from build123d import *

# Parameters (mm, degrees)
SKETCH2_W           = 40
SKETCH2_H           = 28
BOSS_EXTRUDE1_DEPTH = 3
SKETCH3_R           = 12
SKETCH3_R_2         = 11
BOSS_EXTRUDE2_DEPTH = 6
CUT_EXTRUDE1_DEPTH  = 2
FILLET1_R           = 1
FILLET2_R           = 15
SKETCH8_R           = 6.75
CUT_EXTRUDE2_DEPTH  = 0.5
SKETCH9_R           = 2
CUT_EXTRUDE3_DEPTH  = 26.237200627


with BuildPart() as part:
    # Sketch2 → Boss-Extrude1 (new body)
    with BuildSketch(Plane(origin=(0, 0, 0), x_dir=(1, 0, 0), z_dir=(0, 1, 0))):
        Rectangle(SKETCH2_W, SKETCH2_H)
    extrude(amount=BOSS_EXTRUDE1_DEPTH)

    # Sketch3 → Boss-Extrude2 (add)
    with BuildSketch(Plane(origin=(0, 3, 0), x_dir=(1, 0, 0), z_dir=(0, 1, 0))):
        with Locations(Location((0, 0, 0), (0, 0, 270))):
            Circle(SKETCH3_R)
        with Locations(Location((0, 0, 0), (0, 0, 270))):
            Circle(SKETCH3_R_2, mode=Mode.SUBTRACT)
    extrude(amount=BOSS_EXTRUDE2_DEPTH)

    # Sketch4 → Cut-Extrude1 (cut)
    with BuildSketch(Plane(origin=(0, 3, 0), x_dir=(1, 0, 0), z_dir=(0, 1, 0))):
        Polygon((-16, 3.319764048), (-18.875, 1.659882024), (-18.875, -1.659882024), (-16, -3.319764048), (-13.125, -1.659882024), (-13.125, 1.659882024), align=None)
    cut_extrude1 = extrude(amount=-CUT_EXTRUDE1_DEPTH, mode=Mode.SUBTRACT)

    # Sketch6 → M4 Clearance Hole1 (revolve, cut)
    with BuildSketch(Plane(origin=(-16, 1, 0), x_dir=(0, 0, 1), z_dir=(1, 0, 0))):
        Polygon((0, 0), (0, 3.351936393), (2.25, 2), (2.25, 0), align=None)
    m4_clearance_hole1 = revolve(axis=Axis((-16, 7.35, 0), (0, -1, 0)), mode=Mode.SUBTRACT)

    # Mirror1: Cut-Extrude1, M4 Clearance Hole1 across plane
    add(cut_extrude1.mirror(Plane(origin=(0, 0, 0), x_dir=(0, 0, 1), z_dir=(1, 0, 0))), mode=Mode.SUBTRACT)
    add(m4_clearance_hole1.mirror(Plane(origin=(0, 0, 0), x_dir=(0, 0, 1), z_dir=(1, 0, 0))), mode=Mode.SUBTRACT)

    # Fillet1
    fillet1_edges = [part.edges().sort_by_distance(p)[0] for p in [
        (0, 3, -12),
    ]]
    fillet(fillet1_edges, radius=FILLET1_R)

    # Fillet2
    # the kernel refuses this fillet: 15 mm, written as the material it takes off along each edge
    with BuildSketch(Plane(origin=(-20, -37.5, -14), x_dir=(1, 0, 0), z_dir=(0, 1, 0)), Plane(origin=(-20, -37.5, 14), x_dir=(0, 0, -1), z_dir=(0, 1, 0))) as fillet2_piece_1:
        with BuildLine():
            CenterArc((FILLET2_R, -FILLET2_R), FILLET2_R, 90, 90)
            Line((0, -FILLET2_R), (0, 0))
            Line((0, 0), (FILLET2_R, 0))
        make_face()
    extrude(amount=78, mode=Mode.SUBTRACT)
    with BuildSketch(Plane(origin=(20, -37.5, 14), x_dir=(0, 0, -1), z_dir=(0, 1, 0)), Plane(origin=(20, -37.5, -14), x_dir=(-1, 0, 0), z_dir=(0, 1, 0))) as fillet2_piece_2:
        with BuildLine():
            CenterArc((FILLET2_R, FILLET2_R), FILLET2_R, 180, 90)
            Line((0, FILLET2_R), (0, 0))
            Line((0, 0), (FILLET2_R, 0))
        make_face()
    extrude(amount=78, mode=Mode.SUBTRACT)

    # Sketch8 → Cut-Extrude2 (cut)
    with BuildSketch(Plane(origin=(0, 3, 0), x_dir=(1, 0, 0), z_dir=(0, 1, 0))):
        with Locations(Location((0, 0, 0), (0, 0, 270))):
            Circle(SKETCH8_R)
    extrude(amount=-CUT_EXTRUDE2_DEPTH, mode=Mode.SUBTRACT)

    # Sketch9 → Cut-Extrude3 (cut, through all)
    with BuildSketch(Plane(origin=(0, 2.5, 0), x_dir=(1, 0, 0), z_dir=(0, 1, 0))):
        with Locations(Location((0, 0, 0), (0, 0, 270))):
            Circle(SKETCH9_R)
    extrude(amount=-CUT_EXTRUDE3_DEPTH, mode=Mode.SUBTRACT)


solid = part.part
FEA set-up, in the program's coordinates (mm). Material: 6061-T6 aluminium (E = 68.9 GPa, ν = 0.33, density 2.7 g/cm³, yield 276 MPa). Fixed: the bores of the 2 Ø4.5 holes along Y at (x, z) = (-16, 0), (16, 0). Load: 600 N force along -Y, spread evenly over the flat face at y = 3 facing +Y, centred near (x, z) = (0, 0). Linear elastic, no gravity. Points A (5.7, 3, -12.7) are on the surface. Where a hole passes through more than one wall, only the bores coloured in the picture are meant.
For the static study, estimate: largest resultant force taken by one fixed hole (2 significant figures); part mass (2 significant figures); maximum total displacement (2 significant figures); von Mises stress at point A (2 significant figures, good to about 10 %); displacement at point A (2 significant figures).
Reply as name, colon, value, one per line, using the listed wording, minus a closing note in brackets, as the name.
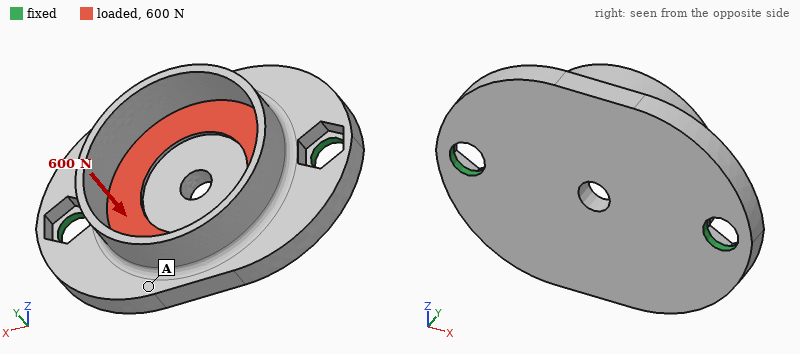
largest resultant force taken by one fixed hole: 450 N
part mass: 8.0 g
maximum total displacement: 44 µm
von Mises stress at point A: 22 MPa
displacement at point A: 31 µm
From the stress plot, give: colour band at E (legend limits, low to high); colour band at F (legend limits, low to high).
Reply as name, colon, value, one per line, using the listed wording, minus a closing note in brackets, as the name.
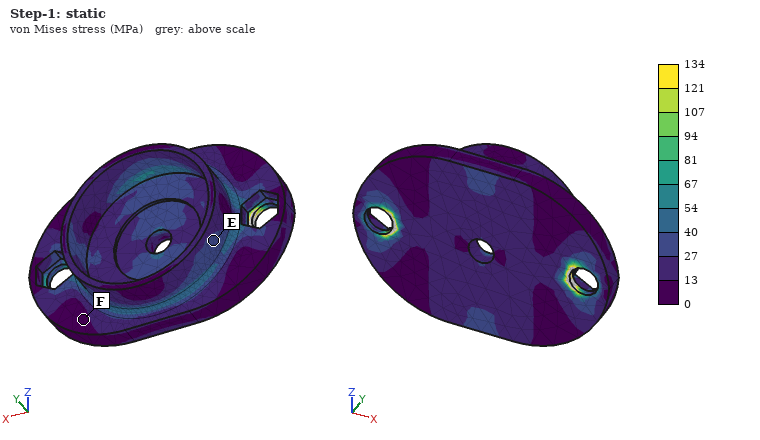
colour band at E: 27 to 40 MPa
colour band at F: 0 to 13 MPa
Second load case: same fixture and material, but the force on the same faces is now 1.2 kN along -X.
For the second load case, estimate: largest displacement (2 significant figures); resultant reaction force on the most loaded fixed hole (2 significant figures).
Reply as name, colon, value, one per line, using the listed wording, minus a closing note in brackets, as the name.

largest displacement: 3.9 µm
resultant reaction force on the most loaded fixed hole: 610 N
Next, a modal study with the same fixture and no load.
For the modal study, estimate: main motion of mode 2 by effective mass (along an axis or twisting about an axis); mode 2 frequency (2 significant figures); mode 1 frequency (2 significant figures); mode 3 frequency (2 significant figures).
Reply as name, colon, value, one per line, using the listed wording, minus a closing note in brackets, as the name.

main motion of mode 2 by effective mass: along Y
mode 2 frequency: 9100 Hz
mode 1 frequency: 5700 Hz
mode 3 frequency: 17 kHz
